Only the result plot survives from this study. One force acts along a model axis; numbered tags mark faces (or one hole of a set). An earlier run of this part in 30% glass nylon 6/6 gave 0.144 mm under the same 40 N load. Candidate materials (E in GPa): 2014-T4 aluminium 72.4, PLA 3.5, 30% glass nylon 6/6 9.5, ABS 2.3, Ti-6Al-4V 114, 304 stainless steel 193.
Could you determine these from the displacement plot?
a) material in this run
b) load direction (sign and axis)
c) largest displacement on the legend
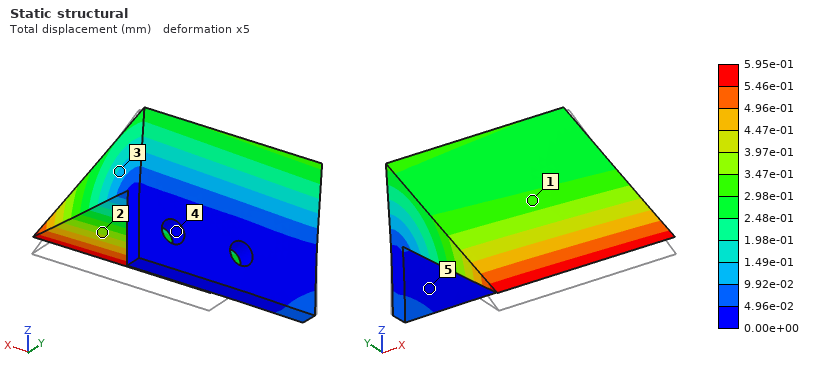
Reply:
ABS
+Z
5.95e-01 mm
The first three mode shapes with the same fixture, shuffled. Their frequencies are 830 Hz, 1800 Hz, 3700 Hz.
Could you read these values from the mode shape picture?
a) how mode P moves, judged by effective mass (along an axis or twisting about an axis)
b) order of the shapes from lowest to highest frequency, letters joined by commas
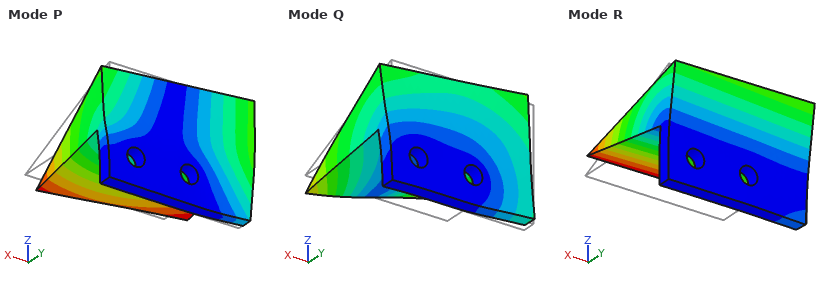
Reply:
along X
R, P, Q
